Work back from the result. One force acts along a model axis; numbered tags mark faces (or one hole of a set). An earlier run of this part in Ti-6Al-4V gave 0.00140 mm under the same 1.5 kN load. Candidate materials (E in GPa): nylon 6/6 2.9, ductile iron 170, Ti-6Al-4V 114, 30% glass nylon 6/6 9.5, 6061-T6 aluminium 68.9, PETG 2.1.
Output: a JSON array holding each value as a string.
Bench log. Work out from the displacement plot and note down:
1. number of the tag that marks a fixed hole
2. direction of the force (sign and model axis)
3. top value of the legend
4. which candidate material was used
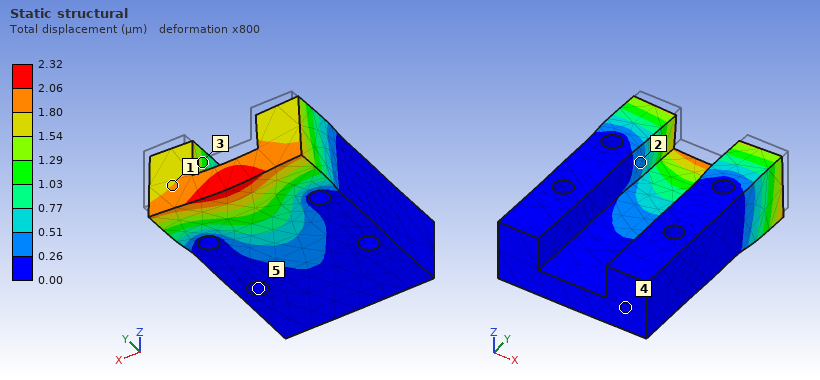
["5", "-Y", "2.32 µm", "6061-T6 aluminium"]
